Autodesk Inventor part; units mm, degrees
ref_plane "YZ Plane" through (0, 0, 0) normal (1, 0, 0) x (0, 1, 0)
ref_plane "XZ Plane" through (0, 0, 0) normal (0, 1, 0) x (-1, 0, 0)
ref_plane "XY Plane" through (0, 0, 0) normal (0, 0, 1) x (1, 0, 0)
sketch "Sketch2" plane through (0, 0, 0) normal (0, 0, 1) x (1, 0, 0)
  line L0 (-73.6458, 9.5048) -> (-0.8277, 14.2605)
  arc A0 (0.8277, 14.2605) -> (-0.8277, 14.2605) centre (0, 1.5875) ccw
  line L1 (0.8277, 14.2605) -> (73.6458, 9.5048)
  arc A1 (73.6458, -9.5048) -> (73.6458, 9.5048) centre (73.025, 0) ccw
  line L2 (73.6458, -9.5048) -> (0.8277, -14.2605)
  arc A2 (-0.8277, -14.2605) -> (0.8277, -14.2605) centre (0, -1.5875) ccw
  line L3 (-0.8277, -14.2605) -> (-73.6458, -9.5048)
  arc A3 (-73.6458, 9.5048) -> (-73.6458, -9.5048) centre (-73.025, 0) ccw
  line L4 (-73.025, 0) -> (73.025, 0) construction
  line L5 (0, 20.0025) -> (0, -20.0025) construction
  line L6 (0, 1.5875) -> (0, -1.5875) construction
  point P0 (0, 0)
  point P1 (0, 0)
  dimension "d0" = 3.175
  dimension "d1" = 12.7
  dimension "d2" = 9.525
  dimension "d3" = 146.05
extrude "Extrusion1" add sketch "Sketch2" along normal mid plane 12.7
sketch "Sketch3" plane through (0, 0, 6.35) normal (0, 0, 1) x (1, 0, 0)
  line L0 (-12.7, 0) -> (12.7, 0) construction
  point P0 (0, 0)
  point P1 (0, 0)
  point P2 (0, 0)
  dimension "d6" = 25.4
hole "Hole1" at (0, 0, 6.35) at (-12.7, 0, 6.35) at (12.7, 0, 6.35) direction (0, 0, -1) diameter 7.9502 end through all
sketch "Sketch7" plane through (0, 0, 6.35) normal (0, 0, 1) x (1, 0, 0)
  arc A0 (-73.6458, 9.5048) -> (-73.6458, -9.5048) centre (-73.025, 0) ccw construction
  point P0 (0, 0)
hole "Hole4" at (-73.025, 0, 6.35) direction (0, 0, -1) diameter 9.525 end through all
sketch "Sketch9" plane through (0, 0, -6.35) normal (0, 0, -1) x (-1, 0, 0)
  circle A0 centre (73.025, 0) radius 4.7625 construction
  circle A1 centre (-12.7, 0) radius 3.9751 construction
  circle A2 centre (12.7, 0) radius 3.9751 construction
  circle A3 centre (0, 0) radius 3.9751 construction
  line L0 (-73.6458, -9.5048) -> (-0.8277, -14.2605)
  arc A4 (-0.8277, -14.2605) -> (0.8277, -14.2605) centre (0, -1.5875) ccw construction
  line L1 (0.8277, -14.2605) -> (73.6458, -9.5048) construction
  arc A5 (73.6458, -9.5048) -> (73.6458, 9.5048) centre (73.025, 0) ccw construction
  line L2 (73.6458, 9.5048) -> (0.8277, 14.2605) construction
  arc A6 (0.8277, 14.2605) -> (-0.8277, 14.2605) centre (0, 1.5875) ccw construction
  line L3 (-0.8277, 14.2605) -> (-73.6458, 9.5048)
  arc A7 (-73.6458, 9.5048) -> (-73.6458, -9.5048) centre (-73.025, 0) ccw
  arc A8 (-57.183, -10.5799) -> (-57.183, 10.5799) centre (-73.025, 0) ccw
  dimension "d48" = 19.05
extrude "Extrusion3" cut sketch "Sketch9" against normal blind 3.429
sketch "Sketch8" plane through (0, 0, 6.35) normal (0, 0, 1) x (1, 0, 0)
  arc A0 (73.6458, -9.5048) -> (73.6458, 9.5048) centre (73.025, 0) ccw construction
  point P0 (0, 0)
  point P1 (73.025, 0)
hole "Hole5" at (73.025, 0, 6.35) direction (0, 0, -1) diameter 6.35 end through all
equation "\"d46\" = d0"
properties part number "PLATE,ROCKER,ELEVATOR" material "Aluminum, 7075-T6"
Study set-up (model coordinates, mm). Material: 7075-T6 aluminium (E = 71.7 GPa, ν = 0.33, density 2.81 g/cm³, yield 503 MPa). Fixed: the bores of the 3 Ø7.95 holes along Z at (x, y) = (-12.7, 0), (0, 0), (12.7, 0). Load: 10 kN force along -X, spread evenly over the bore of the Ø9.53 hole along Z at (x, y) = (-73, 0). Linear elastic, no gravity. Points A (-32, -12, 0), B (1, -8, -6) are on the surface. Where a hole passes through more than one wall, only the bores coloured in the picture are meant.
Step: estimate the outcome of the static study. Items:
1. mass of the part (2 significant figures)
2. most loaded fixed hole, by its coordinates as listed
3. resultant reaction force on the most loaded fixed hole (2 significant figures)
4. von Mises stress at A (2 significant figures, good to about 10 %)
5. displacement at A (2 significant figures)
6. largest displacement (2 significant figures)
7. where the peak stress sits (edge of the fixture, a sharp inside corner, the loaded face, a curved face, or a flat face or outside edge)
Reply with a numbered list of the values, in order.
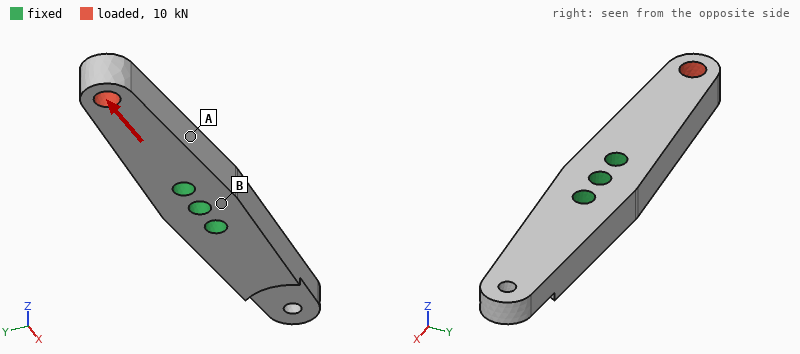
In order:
1. 120 g
2. (-12.7, 0)
3. 8.1 kN
4. 30 MPa
5. 8.9 µm
6. 42 µm
7. the loaded face
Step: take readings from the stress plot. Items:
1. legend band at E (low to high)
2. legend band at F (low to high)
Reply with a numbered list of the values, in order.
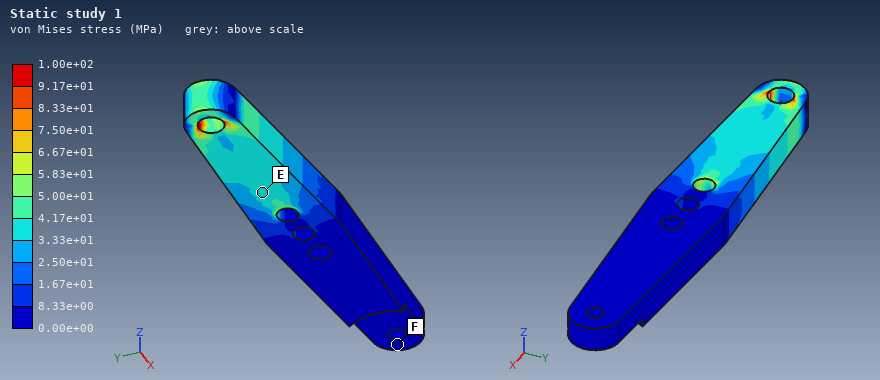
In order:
1. 3.33e+01 to 4.17e+01 MPa
2. 0.00e+00 to 8.33e+00 MPa
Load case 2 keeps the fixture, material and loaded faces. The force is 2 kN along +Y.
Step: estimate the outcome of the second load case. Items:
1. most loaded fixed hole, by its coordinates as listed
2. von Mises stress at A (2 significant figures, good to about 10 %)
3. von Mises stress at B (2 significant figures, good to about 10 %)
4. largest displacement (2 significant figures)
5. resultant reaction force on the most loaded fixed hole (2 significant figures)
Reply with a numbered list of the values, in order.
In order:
1. (-12.7, 0)
2. 66 MPa
3. 16 MPa
4. 0.22 mm
5. 5.2 kN
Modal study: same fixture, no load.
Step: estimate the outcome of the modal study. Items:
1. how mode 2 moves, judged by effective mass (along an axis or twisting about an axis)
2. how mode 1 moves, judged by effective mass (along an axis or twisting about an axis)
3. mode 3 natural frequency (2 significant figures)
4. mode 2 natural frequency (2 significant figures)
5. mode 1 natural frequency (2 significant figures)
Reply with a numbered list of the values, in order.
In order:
1. along Z
2. along Z
3. 4300 Hz
4. 2900 Hz
5. 2700 Hz
